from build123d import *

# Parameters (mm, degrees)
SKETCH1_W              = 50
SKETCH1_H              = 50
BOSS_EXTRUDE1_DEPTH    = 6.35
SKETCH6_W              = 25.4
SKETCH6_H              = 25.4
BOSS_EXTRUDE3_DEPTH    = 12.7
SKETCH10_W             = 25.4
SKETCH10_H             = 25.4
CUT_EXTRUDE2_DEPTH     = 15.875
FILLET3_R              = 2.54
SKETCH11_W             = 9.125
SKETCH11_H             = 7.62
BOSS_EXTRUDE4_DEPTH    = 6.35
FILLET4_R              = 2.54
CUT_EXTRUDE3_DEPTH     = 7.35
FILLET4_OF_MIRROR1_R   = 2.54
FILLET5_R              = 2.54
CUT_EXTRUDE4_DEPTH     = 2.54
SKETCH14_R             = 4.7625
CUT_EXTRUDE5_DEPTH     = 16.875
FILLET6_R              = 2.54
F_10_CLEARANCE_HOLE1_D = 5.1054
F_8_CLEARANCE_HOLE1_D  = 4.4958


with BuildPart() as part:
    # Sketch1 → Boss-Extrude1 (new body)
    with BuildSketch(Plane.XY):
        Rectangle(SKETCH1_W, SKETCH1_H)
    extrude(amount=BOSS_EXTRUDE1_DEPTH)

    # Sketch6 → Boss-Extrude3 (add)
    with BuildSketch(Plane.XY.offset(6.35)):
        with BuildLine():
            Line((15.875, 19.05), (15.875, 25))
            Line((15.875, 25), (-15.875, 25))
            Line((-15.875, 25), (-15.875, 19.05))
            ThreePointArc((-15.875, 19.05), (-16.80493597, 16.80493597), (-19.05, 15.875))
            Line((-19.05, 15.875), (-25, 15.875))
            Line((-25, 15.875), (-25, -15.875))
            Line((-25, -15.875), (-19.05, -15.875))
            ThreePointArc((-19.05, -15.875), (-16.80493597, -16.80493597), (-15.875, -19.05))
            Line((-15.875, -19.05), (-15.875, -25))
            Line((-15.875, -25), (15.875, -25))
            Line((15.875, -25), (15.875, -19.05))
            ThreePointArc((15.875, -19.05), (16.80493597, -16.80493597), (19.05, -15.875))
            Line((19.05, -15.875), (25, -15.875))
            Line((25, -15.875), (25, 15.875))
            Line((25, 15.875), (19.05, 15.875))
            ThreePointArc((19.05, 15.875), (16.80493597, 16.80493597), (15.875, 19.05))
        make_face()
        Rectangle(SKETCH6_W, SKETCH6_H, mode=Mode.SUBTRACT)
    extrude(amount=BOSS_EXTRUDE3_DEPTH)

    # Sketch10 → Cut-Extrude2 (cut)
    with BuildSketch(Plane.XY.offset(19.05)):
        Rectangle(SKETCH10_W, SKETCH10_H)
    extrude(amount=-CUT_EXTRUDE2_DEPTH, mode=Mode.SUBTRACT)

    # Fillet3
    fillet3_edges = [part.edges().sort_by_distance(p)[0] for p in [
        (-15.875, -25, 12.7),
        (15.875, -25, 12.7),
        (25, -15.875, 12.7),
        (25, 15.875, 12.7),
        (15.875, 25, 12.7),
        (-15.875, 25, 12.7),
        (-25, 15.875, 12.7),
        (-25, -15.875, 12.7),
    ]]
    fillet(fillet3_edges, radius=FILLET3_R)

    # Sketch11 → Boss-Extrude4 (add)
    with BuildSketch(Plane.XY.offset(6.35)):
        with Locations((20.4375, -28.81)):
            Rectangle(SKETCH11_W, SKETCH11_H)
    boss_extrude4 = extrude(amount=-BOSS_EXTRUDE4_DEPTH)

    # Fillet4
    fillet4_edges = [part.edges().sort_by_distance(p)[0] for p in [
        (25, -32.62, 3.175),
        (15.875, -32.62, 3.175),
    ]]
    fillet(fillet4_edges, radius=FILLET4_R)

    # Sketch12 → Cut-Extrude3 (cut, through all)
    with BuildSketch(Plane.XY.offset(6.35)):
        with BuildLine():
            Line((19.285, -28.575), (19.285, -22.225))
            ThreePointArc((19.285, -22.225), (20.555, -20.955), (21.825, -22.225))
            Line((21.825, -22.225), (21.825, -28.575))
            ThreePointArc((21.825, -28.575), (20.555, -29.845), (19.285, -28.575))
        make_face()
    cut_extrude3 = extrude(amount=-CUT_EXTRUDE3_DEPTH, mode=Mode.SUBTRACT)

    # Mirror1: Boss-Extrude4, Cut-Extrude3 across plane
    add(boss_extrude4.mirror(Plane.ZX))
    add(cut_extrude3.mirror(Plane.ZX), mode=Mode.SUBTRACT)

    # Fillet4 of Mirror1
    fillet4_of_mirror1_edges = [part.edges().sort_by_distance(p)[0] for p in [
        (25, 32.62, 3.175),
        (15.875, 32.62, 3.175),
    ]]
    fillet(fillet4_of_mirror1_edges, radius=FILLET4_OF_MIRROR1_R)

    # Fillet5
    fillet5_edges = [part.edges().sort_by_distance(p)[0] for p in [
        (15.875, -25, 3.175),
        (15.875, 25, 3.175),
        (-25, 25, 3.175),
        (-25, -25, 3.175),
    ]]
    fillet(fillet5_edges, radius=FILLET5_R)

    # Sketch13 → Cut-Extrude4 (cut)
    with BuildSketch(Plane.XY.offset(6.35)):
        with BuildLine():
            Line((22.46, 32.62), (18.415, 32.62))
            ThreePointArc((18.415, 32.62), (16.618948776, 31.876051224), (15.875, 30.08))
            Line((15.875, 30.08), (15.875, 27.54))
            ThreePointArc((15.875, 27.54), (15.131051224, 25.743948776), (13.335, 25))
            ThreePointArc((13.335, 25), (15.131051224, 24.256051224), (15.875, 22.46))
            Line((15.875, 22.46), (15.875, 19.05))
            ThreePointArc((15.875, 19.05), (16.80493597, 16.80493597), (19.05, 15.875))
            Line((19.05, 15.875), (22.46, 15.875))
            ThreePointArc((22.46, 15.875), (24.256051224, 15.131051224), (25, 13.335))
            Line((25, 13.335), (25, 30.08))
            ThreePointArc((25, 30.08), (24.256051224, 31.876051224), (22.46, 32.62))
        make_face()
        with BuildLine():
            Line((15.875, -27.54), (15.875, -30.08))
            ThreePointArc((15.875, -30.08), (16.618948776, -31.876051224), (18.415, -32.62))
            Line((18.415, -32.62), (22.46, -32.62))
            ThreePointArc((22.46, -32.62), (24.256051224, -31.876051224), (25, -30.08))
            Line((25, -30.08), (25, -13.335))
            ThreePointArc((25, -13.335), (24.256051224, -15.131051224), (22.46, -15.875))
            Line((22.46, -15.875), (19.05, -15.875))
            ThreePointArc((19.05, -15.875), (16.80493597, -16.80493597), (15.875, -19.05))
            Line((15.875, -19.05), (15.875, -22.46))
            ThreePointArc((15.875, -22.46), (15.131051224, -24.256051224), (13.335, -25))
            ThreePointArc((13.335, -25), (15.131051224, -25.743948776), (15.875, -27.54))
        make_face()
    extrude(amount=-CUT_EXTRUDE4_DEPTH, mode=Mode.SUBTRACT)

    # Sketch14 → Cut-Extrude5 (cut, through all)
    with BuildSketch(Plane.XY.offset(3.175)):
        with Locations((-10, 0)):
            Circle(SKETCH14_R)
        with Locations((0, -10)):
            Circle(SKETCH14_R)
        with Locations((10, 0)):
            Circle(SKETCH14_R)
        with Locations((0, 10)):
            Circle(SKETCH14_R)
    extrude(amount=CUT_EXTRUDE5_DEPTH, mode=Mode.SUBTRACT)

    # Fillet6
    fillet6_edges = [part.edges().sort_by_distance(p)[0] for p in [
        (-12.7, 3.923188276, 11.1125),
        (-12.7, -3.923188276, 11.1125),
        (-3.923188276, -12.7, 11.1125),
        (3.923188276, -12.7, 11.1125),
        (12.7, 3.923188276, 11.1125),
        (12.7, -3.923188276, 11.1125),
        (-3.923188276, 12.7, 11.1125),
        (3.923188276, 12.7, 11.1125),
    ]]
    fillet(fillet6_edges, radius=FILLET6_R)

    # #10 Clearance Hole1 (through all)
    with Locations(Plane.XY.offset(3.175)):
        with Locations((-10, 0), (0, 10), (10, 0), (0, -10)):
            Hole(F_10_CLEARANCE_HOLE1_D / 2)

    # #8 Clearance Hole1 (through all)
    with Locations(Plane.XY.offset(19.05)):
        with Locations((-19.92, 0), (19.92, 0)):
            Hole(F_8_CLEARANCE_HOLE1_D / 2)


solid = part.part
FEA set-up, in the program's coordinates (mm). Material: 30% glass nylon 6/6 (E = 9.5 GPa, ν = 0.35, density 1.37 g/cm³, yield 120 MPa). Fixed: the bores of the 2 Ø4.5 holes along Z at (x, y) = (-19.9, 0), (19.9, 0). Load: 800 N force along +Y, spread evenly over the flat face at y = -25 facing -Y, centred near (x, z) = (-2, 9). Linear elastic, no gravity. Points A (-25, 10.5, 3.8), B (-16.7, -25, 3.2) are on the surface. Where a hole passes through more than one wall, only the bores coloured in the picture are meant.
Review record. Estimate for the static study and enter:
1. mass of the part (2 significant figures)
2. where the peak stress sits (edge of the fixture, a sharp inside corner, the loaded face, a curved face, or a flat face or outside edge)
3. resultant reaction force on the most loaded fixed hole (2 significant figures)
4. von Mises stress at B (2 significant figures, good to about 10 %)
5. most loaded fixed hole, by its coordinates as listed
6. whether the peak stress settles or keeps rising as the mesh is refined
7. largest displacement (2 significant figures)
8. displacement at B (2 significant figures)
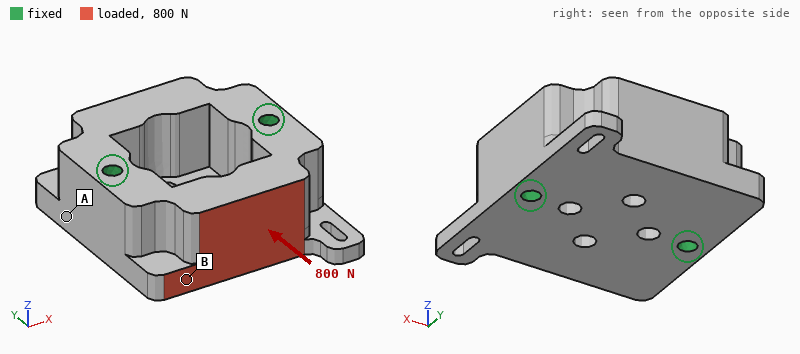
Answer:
43 g
a sharp inside corner
460 N
1.4 MPa
(-19.9, 0)
keeps rising
15 µm
4.8 µm
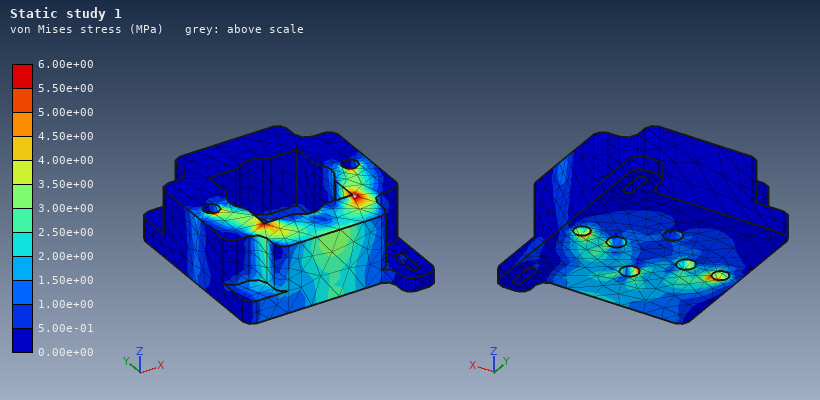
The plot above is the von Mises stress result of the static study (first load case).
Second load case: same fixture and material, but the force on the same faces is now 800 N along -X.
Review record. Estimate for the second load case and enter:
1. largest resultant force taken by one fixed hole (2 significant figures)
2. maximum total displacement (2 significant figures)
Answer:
580 N
22 µm
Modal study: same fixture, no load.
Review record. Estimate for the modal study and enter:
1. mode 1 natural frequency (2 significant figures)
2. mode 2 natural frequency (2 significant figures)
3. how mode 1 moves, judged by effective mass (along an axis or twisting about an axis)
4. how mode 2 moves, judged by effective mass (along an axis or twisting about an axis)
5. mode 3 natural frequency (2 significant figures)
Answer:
6500 Hz
7000 Hz
twisting about X
along Z
8500 Hz
